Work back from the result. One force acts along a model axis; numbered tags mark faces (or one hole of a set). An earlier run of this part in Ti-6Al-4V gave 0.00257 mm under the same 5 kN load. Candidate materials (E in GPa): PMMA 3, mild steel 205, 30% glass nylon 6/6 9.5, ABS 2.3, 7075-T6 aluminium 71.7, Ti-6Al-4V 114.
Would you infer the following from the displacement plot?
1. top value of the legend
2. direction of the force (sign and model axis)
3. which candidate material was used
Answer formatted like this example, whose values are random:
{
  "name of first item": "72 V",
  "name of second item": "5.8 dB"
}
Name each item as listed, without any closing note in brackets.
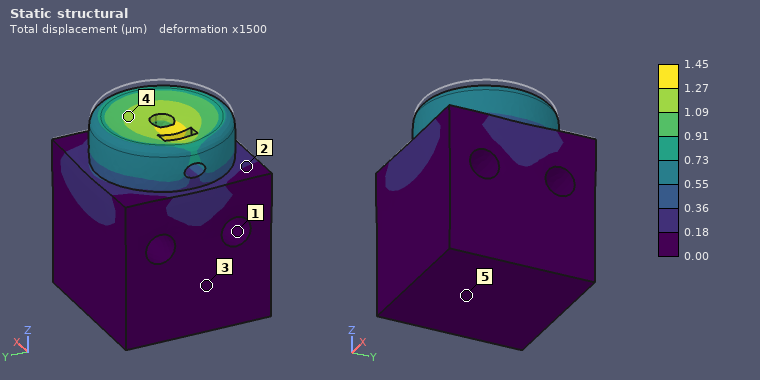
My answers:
{
  "top value of the legend": "1.45 µm",
  "direction of the force": "-Z",
  "which candidate material was used": "mild steel"
}
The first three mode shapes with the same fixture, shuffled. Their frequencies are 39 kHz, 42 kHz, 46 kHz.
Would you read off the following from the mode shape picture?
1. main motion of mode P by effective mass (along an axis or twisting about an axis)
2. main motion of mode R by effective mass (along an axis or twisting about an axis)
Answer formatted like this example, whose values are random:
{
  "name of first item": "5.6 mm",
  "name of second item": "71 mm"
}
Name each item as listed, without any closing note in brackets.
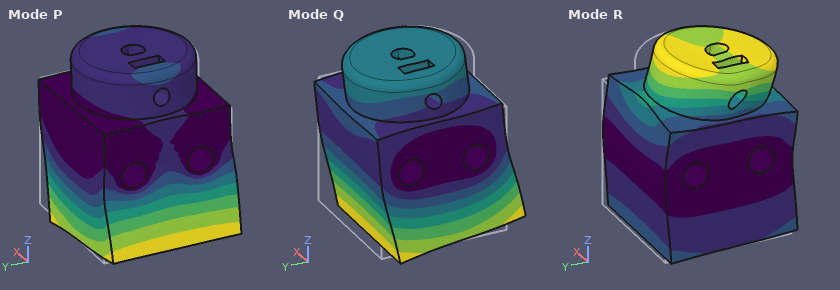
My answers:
{
  "main motion of mode P by effective mass": "along X",
  "main motion of mode R by effective mass": "along Y"
}
